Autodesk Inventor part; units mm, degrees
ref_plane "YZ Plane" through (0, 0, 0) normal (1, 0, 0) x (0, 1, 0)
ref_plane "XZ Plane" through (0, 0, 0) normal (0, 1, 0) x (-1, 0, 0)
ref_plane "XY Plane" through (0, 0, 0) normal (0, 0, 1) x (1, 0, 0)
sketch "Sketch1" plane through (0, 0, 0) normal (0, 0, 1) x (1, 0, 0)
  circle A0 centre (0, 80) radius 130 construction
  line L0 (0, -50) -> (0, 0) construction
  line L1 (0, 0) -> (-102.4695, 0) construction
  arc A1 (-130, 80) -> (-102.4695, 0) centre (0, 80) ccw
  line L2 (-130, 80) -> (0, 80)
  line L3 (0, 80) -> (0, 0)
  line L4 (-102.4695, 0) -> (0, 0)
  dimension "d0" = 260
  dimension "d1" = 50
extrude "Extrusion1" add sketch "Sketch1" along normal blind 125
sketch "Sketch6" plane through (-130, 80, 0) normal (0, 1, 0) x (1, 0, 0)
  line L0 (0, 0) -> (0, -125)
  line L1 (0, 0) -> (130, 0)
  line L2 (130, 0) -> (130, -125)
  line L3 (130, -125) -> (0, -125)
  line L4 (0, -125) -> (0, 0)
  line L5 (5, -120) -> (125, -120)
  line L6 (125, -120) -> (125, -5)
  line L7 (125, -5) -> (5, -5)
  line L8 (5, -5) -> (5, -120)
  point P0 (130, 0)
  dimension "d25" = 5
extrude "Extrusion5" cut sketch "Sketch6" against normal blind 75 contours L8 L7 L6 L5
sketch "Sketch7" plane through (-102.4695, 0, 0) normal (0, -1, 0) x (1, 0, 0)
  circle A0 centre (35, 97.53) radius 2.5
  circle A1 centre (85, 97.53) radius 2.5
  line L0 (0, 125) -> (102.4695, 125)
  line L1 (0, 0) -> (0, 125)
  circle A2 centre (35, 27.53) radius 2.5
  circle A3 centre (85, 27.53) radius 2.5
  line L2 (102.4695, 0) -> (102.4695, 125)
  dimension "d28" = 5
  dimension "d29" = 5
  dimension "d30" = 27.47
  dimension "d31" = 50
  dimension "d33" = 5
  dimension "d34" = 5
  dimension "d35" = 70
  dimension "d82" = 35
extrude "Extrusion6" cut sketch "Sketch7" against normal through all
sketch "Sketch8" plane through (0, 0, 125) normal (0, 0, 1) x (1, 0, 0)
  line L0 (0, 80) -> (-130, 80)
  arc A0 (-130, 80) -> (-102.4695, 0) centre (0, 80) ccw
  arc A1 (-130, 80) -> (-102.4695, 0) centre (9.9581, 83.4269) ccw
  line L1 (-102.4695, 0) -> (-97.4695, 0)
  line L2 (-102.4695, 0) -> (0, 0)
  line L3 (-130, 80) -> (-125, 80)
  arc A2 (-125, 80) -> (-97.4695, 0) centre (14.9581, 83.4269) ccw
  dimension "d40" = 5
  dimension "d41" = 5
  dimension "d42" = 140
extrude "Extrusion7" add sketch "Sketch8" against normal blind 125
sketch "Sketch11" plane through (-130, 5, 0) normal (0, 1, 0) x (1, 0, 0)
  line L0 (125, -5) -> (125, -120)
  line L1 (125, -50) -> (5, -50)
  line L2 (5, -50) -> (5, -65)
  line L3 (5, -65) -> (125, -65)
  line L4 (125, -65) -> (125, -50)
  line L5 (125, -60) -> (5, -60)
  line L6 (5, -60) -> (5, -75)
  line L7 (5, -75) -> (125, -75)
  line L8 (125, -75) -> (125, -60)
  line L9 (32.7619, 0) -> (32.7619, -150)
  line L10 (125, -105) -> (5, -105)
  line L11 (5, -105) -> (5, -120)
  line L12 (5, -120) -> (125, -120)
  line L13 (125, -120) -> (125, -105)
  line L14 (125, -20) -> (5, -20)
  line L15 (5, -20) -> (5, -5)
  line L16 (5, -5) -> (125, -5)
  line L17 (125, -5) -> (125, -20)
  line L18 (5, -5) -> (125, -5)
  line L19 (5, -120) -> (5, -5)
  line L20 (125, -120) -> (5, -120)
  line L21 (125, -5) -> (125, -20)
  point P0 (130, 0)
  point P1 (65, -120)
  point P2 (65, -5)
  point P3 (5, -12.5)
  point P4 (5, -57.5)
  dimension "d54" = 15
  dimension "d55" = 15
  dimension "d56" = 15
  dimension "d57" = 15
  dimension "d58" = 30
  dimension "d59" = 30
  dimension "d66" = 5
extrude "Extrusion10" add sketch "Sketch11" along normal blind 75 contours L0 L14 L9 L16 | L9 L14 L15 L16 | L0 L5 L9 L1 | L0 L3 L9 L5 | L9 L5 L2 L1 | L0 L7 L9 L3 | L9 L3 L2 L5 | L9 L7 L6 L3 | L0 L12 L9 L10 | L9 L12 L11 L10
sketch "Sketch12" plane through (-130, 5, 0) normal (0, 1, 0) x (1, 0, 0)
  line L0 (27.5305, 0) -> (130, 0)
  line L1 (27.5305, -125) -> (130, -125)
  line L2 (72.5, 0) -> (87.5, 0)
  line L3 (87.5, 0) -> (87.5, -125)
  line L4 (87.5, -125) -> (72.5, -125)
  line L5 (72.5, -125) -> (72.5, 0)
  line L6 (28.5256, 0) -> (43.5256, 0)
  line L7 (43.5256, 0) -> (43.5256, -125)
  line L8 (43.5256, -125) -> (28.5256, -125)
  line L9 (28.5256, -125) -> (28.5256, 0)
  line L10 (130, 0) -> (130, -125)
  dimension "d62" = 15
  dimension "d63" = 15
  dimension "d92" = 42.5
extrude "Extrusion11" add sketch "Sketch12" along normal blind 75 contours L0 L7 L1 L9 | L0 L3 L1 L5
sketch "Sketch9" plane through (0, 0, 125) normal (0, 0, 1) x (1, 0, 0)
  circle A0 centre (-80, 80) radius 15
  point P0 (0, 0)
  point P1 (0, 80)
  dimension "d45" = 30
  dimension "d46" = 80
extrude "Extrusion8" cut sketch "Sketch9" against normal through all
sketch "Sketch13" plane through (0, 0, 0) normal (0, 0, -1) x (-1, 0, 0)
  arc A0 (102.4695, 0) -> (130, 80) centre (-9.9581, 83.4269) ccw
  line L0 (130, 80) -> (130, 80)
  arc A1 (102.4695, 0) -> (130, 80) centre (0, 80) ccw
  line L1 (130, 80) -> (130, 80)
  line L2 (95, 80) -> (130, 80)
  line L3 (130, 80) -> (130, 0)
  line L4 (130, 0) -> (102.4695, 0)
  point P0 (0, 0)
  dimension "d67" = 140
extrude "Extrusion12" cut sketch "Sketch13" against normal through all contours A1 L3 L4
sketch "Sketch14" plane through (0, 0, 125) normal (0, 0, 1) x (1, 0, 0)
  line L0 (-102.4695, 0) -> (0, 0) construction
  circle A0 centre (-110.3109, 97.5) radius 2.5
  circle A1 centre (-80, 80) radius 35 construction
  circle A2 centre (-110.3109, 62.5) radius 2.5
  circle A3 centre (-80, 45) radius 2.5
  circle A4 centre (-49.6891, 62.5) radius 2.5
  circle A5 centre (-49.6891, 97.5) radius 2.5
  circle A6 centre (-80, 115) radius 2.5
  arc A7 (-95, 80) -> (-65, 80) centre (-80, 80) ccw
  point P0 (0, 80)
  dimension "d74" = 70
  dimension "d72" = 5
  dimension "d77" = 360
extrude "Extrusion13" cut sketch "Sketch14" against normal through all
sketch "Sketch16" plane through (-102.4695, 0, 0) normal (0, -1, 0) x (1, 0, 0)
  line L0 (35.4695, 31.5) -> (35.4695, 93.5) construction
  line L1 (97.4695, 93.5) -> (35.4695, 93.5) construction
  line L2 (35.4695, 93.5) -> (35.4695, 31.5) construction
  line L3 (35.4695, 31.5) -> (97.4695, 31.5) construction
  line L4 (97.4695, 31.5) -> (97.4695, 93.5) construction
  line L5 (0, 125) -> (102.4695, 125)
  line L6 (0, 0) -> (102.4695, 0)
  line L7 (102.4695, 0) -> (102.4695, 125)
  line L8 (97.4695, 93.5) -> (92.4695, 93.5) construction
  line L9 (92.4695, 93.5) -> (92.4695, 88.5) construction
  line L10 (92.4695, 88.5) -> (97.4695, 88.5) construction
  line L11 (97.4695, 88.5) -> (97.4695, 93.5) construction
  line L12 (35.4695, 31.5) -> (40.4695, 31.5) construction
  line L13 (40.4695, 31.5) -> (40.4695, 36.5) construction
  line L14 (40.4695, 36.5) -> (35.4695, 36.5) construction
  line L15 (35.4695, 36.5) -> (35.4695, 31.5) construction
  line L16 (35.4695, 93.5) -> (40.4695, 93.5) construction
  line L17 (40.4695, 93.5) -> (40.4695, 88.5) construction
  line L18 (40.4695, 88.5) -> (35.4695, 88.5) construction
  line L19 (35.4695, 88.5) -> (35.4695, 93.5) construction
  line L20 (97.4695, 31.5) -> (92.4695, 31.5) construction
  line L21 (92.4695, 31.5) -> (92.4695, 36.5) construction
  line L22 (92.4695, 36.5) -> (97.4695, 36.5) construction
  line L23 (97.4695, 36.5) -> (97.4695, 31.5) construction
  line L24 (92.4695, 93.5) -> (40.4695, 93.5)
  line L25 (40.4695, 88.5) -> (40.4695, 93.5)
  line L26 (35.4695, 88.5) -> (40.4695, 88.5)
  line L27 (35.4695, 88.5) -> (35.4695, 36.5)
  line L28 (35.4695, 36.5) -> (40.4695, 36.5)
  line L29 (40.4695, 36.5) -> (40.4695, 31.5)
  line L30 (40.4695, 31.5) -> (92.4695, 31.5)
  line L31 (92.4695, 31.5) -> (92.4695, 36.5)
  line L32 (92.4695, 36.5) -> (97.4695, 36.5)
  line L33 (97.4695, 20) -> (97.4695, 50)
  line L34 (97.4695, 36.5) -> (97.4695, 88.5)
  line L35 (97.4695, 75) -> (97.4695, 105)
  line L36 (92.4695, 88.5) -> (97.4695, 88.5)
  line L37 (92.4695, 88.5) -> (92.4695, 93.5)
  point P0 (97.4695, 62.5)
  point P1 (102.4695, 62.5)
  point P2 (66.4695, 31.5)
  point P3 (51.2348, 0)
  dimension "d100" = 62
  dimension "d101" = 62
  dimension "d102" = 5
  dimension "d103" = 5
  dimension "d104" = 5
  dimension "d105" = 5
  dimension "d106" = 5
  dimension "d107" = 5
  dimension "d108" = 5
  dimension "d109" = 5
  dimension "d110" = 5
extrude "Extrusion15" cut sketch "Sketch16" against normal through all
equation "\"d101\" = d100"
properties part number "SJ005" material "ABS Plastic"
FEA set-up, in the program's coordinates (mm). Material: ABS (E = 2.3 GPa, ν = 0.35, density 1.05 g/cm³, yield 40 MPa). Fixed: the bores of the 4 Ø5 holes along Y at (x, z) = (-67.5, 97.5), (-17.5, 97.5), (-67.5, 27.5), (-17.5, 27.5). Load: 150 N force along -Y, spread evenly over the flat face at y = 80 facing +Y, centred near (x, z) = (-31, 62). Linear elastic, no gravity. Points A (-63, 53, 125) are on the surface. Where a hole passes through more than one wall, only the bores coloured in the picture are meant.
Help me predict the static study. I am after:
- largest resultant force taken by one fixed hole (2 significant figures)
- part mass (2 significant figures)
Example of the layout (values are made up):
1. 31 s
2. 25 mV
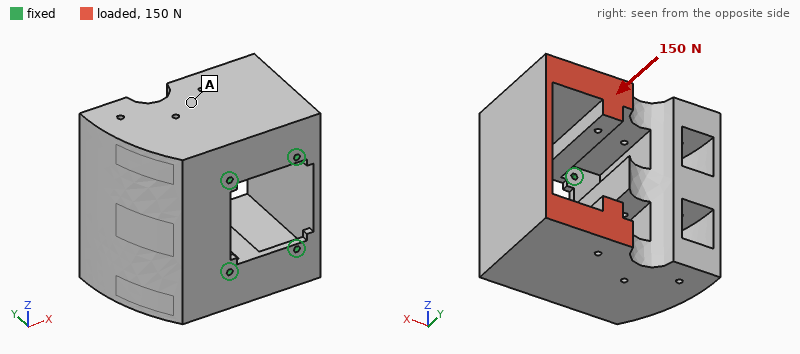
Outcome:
1. 55 N
2. 670 g
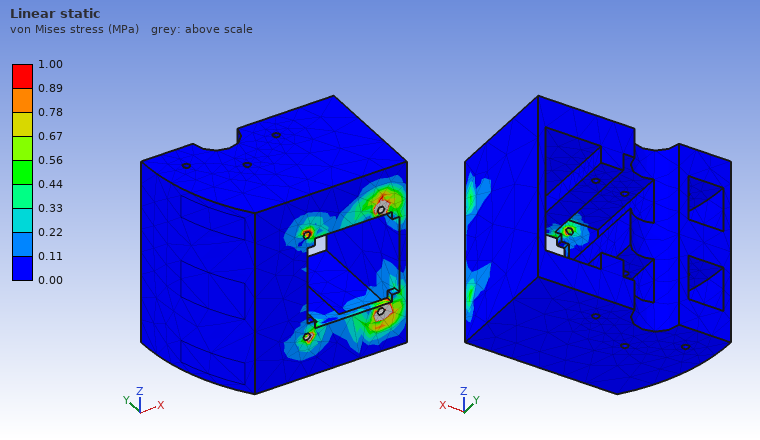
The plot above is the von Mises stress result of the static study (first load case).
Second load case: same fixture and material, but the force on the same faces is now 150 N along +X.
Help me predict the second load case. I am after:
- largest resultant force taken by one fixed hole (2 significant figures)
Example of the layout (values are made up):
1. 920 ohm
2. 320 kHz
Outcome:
1. 120 N
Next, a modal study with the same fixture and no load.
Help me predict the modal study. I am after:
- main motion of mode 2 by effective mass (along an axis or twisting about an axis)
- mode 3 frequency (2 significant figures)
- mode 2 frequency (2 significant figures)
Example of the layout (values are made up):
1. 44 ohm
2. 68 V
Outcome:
1. along Z
2. 780 Hz
3. 410 Hz
